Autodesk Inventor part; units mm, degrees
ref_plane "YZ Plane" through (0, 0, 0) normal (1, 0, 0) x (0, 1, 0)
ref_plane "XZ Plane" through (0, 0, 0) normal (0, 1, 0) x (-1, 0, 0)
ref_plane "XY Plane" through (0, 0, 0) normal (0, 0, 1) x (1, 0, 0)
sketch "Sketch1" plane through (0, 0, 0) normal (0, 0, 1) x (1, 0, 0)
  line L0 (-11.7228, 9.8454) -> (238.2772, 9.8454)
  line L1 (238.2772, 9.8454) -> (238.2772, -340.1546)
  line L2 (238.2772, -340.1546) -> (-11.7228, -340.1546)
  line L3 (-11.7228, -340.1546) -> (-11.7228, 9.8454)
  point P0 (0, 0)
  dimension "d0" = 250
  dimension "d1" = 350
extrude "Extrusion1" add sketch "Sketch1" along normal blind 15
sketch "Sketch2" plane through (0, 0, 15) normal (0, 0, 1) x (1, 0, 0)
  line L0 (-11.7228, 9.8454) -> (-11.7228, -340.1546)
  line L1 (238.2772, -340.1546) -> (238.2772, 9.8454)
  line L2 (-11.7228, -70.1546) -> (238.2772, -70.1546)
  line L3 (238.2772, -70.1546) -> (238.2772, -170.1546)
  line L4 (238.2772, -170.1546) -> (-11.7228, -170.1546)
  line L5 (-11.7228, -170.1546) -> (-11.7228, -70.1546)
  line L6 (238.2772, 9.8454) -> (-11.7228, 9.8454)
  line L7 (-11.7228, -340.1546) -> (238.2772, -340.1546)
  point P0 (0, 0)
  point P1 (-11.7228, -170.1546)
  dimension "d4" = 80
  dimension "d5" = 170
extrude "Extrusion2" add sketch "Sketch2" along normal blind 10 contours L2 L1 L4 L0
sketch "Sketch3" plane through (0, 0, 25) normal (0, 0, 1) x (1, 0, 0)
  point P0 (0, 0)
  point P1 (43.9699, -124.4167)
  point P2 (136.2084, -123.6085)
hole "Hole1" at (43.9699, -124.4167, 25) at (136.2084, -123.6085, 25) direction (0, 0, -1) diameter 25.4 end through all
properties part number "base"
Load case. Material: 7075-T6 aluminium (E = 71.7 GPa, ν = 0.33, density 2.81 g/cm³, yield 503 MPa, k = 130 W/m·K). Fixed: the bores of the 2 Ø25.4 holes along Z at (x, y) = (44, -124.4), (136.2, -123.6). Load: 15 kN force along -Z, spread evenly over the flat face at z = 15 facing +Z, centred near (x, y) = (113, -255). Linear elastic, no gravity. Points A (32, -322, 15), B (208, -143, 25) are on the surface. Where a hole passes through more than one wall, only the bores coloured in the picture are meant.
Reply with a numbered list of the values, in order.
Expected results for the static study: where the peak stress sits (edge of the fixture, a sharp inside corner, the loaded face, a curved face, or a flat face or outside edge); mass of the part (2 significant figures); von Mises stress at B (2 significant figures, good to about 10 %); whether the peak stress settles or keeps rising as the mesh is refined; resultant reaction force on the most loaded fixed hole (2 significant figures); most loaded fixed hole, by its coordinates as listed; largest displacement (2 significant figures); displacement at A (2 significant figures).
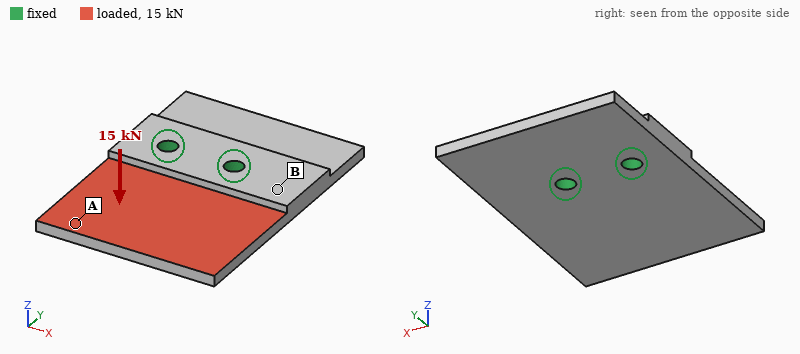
1. edge of the fixture
2. 4.3 kg
3. 41 MPa
4. keeps rising
5. 9.5 kN
6. (136.2, -123.6)
7. 2.6 mm
8. 2.2 mm
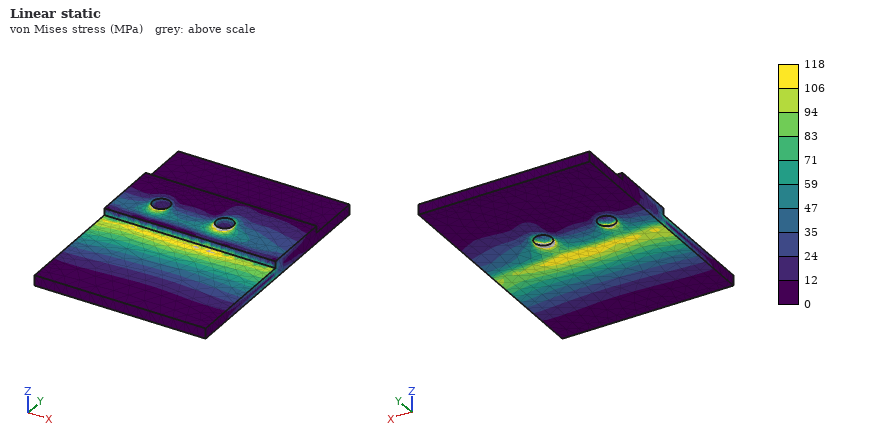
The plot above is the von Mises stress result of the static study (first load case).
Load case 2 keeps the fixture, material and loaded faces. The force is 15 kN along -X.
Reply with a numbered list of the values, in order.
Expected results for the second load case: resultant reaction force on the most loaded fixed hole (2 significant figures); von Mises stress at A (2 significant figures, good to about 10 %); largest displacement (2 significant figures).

1. 19 kN
2. 3.5 MPa
3. 0.17 mm
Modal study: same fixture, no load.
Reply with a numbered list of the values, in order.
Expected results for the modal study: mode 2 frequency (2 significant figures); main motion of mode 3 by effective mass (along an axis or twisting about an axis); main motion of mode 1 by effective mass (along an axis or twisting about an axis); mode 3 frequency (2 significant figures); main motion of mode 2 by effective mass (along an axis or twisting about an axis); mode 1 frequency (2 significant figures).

1. 650 Hz
2. along Z
3. along Z
4. 1100 Hz
5. twisting about Y
6. 360 Hz
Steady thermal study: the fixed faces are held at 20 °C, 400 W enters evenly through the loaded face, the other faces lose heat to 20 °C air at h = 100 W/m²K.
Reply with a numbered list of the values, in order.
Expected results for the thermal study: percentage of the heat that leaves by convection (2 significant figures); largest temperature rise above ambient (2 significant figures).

1. 56 %
2. 46 K
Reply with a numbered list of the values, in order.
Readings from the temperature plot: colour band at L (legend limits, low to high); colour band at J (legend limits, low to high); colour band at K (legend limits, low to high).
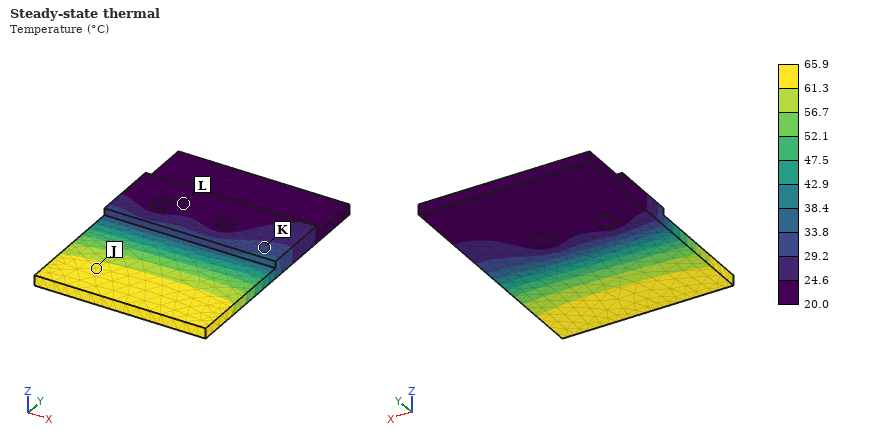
1. 20.0 to 24.6 °C
2. 61.3 to 65.9 °C
3. 29.2 to 33.8 °C
